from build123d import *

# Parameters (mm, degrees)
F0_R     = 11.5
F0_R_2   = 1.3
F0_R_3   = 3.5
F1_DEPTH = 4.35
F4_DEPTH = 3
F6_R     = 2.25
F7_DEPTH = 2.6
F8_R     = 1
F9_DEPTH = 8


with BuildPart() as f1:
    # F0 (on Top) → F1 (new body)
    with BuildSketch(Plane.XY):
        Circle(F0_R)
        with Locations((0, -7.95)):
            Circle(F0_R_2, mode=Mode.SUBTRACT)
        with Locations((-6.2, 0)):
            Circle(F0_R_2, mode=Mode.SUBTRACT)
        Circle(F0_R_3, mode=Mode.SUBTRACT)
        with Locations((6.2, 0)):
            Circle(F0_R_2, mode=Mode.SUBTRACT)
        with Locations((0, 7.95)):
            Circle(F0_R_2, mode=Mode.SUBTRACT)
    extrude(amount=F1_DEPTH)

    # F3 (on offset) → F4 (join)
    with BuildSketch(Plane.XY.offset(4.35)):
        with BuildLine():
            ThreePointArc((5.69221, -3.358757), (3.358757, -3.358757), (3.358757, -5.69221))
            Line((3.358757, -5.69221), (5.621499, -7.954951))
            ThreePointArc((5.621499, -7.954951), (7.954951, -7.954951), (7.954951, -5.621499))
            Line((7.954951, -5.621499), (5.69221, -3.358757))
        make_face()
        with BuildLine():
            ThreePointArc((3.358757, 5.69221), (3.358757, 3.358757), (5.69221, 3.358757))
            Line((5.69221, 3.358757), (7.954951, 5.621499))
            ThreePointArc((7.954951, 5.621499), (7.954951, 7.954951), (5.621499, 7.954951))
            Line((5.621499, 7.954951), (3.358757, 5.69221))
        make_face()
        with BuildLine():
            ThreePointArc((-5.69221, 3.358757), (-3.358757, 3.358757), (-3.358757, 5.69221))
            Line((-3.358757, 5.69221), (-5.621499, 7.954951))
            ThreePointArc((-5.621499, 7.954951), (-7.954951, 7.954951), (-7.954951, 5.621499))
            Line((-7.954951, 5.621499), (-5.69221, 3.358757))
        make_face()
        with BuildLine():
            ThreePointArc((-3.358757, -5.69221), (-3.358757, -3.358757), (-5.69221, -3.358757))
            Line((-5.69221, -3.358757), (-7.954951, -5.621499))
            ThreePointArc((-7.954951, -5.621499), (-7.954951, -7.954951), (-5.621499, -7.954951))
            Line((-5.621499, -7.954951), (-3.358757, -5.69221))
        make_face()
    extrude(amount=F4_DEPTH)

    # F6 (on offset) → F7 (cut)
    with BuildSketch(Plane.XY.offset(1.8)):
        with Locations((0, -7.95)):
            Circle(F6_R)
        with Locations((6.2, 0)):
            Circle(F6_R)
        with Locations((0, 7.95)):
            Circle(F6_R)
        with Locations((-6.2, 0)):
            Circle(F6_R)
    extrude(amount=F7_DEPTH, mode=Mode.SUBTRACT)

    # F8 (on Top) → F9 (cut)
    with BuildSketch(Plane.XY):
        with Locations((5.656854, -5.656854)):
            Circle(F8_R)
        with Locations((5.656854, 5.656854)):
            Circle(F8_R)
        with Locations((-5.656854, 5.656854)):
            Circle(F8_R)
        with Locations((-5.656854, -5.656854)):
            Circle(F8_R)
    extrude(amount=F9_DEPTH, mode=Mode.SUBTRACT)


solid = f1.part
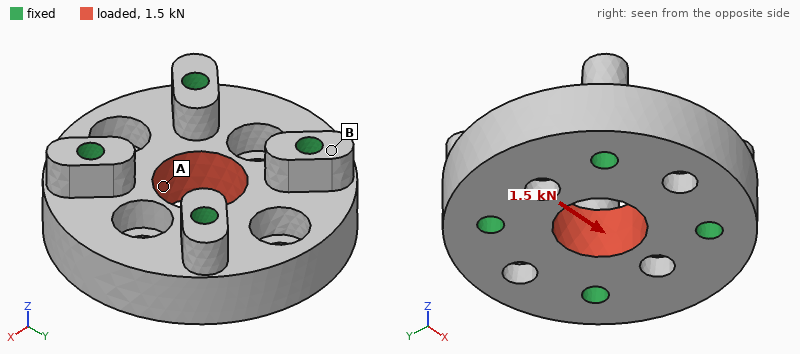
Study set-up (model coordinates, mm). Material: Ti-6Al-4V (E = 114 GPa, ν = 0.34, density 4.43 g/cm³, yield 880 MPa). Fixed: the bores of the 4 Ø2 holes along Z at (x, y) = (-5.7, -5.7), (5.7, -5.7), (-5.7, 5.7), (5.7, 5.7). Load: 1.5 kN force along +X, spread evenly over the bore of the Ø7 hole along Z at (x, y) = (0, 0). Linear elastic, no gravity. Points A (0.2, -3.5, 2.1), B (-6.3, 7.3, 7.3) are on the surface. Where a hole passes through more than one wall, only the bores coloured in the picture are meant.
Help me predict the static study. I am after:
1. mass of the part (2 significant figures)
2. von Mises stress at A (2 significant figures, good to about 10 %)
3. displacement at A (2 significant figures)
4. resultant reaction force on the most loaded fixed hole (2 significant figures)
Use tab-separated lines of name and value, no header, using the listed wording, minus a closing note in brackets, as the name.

mass of the part	7.0 g
von Mises stress at A	29 MPa
displacement at A	0.74 µm
resultant reaction force on the most loaded fixed hole	390 N
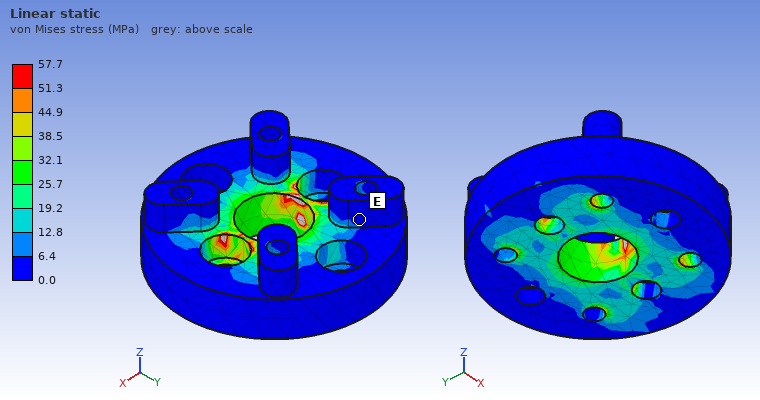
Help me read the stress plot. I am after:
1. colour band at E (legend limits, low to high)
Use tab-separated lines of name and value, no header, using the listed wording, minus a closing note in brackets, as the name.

colour band at E	0.0 to 6.4 MPa
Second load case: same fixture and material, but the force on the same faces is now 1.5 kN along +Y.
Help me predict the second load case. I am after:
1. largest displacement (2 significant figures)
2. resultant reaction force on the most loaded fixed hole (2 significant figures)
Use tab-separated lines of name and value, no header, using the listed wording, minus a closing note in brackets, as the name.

largest displacement	1.6 µm
resultant reaction force on the most loaded fixed hole	390 N
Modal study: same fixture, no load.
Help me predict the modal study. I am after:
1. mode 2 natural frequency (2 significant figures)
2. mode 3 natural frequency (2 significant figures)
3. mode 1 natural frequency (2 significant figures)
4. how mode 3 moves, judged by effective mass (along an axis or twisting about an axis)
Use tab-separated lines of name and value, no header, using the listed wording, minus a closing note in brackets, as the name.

mode 2 natural frequency	81 kHz
mode 3 natural frequency	84 kHz
mode 1 natural frequency	79 kHz
how mode 3 moves, judged by effective mass	twisting about X
